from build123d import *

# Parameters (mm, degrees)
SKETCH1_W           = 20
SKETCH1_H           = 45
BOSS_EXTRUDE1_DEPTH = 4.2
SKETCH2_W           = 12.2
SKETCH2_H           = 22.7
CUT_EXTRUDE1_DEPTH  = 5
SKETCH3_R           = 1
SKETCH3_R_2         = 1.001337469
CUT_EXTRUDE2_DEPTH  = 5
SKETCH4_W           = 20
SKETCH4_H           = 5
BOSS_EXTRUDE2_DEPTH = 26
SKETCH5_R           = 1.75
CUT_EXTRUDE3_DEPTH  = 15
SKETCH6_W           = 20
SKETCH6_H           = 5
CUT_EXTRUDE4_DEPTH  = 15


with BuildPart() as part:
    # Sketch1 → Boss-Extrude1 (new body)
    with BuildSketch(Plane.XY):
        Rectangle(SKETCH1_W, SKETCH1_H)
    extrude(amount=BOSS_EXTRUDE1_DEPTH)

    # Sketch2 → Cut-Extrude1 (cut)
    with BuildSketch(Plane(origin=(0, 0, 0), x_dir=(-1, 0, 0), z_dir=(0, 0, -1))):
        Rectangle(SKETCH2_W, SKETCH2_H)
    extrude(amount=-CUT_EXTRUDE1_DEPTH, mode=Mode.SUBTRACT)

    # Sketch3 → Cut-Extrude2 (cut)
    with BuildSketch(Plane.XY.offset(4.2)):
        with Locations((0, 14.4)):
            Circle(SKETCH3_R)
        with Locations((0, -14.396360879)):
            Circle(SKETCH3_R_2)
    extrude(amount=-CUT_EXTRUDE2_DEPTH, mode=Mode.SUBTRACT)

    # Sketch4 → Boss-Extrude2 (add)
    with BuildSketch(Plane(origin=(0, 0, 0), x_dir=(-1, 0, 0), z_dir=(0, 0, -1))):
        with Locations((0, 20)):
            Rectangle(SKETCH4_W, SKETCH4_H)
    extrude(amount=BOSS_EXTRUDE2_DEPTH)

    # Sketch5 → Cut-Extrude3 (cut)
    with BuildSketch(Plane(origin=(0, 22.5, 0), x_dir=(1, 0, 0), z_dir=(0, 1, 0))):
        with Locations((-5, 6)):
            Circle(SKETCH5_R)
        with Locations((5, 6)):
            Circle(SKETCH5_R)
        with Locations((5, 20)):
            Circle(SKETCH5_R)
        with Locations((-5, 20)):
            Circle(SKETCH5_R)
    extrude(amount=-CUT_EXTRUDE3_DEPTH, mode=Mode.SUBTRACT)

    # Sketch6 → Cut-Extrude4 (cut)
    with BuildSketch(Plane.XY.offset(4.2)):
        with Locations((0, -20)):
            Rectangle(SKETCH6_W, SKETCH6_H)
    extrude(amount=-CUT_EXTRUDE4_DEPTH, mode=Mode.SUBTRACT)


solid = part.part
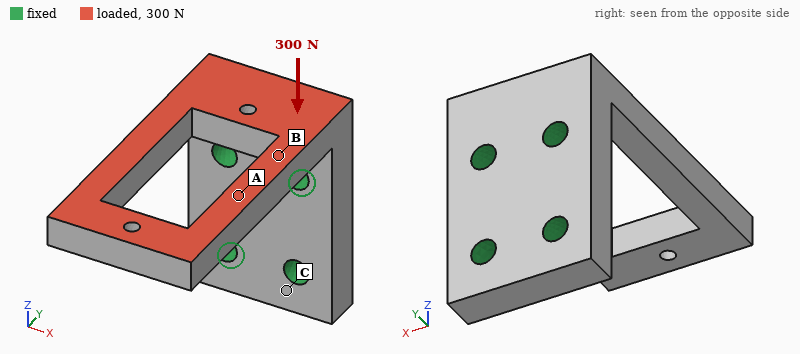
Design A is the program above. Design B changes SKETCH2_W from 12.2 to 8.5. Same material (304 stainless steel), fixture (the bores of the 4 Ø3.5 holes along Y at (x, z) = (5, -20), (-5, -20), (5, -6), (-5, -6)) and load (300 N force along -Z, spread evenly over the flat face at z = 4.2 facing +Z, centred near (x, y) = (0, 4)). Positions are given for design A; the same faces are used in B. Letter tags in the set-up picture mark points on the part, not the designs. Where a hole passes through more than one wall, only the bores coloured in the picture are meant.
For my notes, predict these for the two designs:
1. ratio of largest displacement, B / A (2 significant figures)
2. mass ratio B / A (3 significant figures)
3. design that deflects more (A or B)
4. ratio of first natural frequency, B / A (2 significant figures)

0.80
1.08
A
1.1
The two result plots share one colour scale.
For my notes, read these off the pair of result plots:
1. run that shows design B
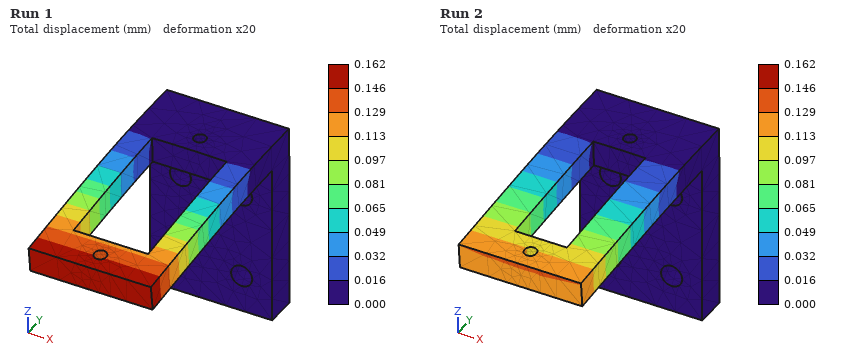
Run 2
